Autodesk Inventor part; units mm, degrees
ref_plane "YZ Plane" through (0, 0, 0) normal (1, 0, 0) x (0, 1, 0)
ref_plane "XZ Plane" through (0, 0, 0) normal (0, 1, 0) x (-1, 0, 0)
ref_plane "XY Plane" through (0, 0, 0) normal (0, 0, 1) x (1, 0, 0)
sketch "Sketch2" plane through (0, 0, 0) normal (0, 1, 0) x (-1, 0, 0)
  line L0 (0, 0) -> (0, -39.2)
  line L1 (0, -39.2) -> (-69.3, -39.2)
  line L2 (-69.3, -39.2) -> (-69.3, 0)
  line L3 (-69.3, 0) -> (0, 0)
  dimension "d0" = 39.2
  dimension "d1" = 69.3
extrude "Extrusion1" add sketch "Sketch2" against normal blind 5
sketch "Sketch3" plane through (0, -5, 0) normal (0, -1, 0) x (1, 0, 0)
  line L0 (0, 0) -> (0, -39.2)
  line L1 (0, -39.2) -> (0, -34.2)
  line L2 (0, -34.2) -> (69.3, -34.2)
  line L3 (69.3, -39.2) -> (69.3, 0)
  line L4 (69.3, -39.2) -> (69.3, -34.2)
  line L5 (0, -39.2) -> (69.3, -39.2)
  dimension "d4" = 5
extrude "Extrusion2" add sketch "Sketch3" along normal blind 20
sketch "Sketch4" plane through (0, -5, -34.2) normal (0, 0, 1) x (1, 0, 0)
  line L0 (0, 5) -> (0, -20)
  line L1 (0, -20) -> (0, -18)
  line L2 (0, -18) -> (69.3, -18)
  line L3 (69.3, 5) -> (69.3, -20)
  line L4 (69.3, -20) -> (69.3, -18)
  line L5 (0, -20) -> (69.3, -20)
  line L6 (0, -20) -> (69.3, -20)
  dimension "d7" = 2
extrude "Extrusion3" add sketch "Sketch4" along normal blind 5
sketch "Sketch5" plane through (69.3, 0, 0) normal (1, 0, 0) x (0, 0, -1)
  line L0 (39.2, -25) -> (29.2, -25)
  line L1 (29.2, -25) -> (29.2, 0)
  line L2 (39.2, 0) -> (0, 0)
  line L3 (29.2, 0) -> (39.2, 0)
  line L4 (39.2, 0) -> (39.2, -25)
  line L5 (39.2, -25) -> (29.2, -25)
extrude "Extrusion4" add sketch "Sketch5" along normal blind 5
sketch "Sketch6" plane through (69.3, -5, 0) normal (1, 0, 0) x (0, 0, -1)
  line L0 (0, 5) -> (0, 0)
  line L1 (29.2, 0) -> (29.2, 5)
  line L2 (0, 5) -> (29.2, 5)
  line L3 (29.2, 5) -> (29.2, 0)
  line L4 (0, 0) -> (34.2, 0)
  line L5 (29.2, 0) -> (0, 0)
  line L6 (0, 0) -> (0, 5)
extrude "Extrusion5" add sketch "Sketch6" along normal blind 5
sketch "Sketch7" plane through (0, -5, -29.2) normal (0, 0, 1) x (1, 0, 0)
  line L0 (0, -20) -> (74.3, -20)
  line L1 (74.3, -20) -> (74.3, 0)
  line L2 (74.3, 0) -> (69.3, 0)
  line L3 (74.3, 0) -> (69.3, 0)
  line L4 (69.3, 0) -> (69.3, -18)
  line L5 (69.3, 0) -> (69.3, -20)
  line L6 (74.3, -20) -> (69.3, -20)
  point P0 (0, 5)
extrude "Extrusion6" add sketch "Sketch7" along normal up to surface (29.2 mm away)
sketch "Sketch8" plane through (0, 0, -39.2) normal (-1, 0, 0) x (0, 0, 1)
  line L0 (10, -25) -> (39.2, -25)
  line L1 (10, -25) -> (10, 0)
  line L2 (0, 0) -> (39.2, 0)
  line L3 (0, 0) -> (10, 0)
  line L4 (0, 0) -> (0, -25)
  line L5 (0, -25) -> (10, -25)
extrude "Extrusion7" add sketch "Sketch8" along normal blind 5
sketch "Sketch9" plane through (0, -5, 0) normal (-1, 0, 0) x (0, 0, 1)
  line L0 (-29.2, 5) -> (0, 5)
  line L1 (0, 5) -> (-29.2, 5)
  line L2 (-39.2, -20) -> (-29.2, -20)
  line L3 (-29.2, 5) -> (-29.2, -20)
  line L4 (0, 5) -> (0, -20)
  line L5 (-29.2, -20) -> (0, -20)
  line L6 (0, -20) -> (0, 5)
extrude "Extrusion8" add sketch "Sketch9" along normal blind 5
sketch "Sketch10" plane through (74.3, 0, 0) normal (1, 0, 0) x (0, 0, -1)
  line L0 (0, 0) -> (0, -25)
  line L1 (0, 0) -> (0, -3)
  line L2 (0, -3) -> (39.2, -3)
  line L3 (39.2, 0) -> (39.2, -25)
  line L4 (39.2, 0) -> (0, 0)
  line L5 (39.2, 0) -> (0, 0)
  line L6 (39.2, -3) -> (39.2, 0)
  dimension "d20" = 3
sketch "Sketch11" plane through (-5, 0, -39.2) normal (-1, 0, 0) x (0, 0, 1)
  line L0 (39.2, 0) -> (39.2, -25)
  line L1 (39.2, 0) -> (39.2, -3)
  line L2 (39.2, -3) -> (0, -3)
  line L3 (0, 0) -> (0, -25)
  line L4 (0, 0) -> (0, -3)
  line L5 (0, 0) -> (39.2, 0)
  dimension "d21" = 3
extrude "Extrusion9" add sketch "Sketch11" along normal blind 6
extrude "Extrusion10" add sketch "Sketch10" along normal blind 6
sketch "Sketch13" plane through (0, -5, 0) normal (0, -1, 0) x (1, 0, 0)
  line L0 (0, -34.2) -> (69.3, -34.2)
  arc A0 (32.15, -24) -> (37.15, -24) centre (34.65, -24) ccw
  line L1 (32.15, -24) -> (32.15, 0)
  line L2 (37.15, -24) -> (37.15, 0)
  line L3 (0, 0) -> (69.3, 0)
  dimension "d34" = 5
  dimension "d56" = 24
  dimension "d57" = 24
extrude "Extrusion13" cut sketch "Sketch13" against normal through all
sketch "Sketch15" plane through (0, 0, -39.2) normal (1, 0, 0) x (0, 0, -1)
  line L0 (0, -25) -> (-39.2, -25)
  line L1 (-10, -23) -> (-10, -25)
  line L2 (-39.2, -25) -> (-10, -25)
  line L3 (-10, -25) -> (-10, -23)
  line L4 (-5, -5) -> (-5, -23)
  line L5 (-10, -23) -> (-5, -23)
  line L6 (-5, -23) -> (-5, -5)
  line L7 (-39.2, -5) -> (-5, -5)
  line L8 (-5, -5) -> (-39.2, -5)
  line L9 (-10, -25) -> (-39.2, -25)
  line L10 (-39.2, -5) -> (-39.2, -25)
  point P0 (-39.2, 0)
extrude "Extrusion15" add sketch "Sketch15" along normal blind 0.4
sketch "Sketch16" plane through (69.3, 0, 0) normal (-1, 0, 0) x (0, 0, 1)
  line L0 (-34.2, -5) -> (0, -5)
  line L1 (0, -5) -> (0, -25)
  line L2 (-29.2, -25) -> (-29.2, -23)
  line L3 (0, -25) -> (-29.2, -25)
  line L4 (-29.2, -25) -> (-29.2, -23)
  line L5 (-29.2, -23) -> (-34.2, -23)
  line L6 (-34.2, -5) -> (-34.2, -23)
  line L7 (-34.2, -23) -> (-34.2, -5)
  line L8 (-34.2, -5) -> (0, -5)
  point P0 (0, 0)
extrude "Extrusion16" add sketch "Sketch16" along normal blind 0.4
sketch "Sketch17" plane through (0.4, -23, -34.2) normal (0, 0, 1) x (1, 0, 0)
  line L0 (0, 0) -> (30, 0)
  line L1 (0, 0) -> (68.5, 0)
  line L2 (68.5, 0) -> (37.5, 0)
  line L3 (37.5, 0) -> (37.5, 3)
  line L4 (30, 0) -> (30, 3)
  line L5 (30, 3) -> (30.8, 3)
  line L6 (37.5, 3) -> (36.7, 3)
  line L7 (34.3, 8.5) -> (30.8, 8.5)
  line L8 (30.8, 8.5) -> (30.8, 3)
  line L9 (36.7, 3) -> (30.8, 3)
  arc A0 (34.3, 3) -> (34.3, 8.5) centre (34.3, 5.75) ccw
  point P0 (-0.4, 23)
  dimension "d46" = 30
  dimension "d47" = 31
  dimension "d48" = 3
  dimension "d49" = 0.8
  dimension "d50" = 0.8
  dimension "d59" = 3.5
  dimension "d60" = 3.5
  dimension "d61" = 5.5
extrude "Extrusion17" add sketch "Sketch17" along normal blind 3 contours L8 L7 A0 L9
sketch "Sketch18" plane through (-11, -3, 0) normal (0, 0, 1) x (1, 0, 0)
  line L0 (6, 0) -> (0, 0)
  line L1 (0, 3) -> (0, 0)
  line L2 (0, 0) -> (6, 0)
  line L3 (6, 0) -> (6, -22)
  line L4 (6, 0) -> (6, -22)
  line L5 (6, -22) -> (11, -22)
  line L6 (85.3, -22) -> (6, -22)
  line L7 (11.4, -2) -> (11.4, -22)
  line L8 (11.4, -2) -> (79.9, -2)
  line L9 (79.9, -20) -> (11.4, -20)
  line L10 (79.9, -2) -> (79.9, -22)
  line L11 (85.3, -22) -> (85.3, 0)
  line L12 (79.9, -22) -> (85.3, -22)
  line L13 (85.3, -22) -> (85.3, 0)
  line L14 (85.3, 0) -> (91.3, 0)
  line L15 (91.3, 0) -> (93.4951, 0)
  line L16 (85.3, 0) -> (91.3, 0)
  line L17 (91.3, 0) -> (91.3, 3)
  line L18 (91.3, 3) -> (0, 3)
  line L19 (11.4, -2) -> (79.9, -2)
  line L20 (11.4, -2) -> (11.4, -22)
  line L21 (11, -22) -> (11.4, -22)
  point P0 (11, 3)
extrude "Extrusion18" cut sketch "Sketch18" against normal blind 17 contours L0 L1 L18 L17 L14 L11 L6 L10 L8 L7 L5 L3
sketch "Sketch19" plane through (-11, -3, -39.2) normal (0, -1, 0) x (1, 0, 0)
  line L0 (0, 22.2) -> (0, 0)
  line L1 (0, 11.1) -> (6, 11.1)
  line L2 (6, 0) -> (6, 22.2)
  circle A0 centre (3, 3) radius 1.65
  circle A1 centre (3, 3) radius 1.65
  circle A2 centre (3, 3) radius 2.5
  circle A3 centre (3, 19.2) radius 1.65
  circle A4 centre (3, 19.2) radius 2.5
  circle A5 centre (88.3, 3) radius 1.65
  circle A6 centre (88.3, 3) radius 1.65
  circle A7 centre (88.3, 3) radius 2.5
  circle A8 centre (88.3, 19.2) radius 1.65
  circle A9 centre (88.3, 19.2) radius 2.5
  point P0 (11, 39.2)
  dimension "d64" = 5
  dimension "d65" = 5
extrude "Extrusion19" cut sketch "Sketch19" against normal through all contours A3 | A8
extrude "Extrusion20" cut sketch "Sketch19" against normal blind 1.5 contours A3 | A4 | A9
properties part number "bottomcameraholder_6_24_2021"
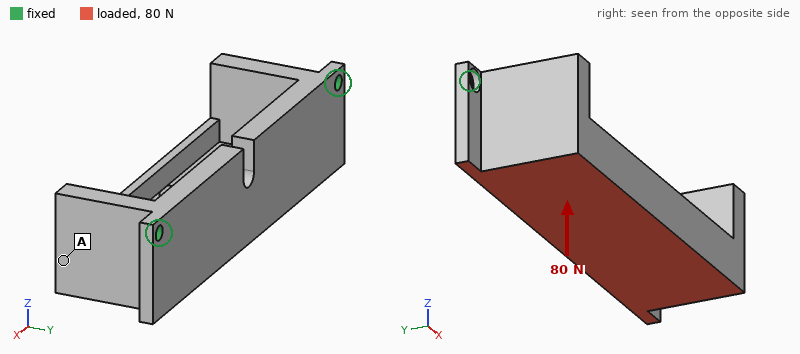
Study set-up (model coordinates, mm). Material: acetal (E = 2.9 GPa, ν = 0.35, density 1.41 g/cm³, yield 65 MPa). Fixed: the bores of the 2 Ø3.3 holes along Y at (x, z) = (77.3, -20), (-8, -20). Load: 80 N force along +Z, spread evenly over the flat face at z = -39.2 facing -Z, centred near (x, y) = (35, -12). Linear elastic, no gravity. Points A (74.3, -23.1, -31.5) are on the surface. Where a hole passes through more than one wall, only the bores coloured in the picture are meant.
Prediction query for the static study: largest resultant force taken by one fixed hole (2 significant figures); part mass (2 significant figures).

55 N
31 g
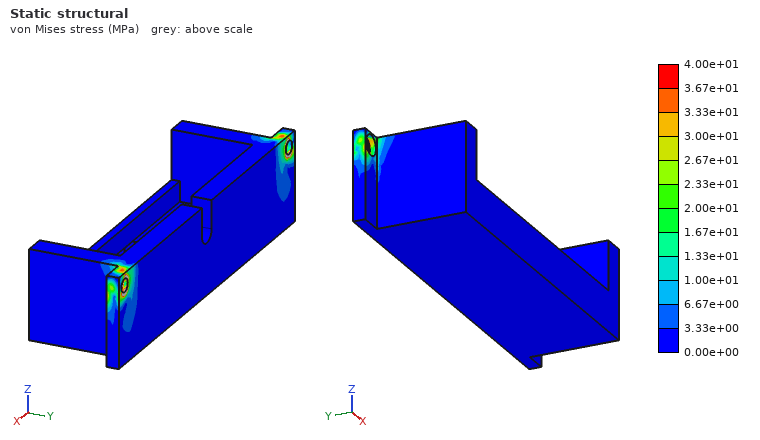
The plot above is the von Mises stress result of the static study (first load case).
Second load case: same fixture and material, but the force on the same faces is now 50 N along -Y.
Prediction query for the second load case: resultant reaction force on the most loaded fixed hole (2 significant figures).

25 N
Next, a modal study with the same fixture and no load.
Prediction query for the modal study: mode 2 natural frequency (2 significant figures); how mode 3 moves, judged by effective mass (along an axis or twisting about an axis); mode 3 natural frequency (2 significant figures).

890 Hz
along Y
1500 Hz
